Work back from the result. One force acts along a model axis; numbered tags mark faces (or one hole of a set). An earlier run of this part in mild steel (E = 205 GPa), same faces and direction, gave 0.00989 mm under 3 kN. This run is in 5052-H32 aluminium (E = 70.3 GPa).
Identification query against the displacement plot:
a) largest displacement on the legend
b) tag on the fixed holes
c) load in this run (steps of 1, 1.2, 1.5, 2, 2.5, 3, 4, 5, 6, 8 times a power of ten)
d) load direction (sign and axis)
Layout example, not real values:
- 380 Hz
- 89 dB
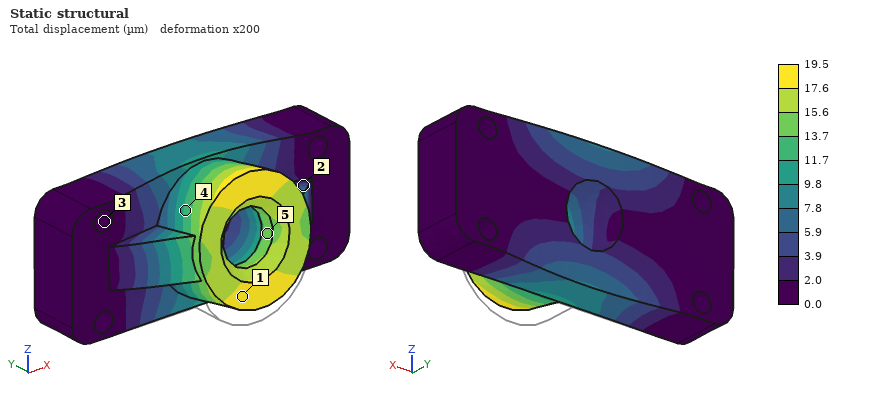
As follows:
- 19.5 µm
- 3
- 2 kN
- +Z
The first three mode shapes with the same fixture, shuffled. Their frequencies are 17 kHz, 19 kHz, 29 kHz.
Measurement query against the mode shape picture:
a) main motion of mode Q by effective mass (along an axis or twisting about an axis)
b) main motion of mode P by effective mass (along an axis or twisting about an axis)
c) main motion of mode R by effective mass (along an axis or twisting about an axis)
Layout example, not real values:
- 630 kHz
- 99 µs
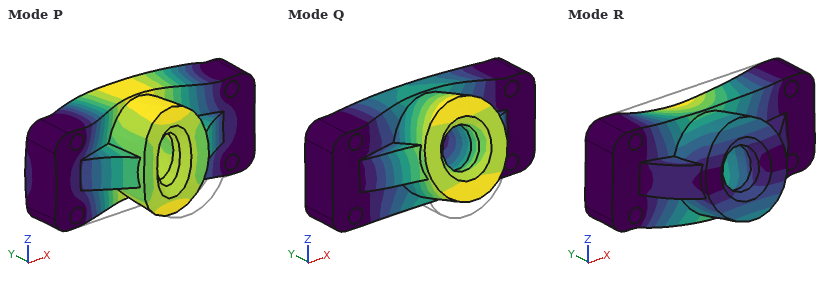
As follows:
- along Z
- along Y
- along Z
